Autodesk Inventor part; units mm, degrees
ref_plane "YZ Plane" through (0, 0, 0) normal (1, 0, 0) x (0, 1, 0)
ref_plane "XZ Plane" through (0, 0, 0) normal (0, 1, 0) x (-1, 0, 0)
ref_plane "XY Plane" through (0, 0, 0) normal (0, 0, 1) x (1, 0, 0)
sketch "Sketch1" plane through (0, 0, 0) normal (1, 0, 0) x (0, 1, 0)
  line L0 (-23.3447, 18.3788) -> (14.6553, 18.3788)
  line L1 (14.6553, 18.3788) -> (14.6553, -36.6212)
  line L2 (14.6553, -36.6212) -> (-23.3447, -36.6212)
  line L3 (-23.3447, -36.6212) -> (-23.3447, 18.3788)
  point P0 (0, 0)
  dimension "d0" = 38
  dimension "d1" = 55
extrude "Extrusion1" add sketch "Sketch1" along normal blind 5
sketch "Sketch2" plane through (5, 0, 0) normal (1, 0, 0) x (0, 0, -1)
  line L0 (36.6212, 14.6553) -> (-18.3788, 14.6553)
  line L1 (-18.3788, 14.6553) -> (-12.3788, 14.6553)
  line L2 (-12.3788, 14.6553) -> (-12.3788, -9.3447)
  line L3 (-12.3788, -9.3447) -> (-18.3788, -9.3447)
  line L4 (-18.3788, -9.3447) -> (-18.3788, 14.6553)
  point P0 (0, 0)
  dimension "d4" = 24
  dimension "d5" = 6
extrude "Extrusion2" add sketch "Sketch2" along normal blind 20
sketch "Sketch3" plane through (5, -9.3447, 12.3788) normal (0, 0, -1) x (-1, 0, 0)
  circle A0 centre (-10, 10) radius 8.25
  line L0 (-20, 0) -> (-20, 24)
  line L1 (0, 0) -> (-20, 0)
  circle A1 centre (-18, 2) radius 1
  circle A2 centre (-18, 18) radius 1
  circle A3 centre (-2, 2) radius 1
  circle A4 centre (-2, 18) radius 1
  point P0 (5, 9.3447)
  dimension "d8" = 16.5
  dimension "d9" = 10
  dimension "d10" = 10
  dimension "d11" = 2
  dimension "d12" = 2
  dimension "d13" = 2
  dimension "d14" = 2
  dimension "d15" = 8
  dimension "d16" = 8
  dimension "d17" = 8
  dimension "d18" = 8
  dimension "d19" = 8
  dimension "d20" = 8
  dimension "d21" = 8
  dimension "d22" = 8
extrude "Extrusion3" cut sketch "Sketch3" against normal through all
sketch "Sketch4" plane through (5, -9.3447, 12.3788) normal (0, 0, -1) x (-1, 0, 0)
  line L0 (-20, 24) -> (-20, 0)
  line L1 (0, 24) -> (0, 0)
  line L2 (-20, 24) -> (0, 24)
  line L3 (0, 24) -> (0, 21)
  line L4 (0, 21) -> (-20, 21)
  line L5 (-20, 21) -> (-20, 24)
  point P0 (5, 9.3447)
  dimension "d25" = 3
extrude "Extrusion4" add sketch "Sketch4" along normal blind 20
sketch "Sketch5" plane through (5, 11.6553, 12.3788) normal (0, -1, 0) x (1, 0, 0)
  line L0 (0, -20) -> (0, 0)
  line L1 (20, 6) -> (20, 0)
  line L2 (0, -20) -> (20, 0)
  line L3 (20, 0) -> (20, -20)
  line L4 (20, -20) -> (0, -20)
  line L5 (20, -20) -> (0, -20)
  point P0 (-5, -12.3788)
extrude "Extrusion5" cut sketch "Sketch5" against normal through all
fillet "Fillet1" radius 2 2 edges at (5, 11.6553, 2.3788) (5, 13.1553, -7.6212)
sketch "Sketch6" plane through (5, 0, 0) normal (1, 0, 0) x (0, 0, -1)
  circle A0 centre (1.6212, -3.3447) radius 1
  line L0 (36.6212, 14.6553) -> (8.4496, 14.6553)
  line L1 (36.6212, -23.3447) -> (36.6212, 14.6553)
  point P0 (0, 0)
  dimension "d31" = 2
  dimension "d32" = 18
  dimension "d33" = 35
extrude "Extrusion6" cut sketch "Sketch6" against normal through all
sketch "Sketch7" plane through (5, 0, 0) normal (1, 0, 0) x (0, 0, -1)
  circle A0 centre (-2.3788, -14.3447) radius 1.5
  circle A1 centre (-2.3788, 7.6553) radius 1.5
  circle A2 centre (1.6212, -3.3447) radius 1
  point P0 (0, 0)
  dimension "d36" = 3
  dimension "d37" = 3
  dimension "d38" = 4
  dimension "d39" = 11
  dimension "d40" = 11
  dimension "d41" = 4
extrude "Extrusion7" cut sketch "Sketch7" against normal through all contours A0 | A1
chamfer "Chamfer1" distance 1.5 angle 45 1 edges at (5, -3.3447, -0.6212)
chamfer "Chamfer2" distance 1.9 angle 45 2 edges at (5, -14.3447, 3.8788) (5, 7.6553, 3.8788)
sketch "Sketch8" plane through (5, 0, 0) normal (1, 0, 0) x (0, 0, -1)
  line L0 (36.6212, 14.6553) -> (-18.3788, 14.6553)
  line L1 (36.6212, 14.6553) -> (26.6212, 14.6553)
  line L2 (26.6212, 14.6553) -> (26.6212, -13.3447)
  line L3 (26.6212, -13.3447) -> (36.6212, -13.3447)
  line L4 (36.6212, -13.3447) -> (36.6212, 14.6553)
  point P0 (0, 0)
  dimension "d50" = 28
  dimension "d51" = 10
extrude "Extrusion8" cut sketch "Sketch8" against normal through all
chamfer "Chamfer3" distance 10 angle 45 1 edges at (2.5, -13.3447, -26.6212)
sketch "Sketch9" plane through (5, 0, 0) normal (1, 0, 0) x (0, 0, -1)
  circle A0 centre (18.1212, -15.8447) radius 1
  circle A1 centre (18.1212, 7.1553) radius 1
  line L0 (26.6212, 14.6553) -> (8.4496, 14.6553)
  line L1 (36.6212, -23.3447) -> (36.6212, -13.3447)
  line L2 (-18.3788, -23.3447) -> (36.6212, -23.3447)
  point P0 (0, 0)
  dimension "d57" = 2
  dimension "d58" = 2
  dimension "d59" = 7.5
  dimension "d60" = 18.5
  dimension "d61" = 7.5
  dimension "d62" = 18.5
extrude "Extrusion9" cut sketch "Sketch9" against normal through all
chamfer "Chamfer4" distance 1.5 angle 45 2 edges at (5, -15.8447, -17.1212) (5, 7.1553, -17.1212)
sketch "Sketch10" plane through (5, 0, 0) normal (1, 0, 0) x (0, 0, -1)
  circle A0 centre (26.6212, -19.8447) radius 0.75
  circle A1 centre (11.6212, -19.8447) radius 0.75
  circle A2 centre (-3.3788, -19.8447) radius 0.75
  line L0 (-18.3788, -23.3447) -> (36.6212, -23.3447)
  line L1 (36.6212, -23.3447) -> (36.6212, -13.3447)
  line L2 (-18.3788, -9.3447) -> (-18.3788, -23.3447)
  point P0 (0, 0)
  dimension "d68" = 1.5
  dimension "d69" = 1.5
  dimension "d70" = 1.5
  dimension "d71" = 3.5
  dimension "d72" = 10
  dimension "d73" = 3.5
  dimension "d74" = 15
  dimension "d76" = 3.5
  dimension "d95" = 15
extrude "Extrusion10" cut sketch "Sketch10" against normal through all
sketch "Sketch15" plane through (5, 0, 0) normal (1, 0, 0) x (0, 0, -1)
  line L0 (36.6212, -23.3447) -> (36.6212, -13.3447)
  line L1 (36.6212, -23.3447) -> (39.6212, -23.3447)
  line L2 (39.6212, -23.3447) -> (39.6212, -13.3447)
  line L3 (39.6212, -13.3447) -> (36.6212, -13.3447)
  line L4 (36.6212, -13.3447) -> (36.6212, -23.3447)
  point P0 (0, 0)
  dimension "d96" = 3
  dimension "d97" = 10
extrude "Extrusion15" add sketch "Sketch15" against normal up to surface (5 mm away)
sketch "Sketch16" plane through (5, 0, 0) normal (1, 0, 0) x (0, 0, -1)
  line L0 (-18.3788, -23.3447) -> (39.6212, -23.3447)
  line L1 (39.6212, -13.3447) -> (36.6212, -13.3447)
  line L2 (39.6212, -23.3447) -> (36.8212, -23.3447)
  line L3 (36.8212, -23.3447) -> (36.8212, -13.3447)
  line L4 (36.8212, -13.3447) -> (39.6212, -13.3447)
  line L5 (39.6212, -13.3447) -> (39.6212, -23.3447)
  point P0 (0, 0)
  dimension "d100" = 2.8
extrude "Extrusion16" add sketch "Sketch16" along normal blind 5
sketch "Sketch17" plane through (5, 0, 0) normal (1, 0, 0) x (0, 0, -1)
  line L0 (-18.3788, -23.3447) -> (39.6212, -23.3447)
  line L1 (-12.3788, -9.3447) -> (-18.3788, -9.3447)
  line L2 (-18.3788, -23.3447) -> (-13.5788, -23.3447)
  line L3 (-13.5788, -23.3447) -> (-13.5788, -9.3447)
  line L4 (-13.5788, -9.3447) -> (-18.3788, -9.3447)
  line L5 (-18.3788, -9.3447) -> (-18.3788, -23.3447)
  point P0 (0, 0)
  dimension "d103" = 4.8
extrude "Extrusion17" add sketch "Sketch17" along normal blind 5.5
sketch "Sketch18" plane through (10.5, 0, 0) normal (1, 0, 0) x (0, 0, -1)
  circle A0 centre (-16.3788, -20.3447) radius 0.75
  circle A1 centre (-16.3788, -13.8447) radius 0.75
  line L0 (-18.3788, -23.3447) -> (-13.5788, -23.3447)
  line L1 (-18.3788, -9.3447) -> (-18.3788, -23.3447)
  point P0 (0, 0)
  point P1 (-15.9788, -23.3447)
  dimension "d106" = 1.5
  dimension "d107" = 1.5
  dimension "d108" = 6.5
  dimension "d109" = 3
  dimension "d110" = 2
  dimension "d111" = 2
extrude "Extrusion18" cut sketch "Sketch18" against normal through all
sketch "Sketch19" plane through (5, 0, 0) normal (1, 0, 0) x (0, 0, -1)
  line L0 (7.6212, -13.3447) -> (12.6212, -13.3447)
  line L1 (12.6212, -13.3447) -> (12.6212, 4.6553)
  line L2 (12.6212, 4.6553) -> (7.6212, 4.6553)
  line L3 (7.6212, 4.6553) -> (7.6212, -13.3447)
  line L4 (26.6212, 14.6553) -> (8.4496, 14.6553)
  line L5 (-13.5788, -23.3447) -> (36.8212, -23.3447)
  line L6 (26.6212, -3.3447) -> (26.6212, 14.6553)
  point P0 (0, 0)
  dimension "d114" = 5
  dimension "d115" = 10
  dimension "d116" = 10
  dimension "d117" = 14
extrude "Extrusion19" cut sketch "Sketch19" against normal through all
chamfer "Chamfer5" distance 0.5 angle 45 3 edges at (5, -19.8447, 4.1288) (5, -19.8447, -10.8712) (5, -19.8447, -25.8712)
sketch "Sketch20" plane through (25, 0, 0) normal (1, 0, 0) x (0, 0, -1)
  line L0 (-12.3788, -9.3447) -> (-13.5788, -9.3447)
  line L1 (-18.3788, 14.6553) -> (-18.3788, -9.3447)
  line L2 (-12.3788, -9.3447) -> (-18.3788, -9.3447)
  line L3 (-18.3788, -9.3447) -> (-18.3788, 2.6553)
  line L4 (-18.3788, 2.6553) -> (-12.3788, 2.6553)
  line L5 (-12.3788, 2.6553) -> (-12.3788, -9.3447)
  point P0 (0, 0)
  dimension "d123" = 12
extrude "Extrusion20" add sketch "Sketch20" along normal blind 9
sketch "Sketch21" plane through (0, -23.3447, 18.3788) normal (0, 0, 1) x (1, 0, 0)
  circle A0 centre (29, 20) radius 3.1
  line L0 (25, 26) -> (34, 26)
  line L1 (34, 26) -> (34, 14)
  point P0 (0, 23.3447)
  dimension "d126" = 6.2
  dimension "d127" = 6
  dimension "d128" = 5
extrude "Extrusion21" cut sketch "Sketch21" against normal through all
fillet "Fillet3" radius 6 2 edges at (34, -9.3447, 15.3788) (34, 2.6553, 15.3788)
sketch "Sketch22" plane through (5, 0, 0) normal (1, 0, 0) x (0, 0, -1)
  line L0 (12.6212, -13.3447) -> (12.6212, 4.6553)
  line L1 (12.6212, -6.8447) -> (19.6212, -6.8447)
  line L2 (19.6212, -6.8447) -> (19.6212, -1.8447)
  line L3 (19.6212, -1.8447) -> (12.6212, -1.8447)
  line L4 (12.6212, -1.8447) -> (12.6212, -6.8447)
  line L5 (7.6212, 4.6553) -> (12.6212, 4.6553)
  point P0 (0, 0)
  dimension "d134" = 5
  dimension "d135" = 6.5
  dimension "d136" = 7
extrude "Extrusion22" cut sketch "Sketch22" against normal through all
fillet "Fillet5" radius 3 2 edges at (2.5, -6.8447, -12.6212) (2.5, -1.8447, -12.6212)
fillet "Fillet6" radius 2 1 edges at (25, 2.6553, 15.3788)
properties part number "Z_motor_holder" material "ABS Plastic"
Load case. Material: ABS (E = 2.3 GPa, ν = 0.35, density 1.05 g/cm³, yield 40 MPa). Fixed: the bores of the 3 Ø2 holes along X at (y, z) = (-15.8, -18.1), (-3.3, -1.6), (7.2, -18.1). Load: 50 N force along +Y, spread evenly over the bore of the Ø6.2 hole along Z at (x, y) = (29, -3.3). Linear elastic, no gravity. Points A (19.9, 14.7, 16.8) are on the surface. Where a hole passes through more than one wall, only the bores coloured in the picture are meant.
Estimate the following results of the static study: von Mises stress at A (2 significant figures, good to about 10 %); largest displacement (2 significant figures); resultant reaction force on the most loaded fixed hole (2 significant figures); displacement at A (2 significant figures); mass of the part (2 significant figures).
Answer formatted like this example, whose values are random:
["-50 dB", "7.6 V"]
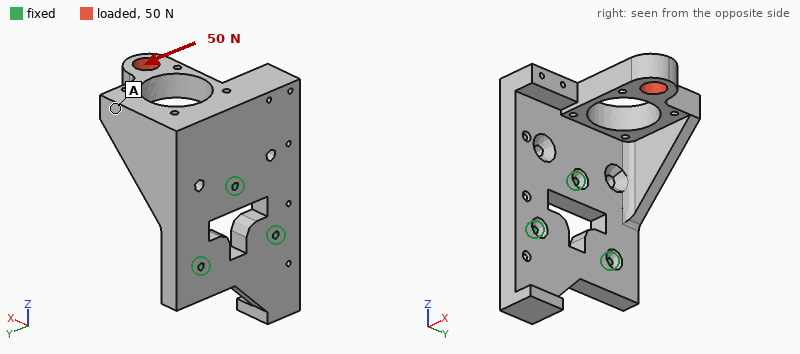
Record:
["1.3 MPa", "0.90 mm", "51 N", "0.69 mm", "12 g"]
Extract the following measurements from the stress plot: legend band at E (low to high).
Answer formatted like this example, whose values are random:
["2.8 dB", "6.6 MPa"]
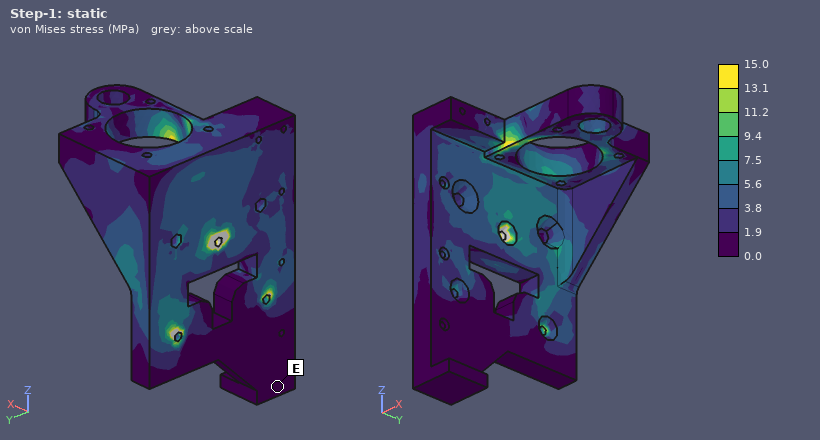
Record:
["0.0 to 1.9 MPa"]
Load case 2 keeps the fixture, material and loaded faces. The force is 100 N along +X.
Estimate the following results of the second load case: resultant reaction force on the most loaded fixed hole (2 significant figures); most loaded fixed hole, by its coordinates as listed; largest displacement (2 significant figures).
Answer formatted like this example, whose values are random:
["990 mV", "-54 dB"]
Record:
["160 N", "(-3.3, -1.6)", "0.79 mm"]
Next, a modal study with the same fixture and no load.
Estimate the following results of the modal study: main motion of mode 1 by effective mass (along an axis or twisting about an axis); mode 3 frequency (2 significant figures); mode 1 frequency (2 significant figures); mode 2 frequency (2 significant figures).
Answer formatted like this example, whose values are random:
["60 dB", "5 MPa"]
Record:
["along X", "2000 Hz", "880 Hz", "1200 Hz"]
